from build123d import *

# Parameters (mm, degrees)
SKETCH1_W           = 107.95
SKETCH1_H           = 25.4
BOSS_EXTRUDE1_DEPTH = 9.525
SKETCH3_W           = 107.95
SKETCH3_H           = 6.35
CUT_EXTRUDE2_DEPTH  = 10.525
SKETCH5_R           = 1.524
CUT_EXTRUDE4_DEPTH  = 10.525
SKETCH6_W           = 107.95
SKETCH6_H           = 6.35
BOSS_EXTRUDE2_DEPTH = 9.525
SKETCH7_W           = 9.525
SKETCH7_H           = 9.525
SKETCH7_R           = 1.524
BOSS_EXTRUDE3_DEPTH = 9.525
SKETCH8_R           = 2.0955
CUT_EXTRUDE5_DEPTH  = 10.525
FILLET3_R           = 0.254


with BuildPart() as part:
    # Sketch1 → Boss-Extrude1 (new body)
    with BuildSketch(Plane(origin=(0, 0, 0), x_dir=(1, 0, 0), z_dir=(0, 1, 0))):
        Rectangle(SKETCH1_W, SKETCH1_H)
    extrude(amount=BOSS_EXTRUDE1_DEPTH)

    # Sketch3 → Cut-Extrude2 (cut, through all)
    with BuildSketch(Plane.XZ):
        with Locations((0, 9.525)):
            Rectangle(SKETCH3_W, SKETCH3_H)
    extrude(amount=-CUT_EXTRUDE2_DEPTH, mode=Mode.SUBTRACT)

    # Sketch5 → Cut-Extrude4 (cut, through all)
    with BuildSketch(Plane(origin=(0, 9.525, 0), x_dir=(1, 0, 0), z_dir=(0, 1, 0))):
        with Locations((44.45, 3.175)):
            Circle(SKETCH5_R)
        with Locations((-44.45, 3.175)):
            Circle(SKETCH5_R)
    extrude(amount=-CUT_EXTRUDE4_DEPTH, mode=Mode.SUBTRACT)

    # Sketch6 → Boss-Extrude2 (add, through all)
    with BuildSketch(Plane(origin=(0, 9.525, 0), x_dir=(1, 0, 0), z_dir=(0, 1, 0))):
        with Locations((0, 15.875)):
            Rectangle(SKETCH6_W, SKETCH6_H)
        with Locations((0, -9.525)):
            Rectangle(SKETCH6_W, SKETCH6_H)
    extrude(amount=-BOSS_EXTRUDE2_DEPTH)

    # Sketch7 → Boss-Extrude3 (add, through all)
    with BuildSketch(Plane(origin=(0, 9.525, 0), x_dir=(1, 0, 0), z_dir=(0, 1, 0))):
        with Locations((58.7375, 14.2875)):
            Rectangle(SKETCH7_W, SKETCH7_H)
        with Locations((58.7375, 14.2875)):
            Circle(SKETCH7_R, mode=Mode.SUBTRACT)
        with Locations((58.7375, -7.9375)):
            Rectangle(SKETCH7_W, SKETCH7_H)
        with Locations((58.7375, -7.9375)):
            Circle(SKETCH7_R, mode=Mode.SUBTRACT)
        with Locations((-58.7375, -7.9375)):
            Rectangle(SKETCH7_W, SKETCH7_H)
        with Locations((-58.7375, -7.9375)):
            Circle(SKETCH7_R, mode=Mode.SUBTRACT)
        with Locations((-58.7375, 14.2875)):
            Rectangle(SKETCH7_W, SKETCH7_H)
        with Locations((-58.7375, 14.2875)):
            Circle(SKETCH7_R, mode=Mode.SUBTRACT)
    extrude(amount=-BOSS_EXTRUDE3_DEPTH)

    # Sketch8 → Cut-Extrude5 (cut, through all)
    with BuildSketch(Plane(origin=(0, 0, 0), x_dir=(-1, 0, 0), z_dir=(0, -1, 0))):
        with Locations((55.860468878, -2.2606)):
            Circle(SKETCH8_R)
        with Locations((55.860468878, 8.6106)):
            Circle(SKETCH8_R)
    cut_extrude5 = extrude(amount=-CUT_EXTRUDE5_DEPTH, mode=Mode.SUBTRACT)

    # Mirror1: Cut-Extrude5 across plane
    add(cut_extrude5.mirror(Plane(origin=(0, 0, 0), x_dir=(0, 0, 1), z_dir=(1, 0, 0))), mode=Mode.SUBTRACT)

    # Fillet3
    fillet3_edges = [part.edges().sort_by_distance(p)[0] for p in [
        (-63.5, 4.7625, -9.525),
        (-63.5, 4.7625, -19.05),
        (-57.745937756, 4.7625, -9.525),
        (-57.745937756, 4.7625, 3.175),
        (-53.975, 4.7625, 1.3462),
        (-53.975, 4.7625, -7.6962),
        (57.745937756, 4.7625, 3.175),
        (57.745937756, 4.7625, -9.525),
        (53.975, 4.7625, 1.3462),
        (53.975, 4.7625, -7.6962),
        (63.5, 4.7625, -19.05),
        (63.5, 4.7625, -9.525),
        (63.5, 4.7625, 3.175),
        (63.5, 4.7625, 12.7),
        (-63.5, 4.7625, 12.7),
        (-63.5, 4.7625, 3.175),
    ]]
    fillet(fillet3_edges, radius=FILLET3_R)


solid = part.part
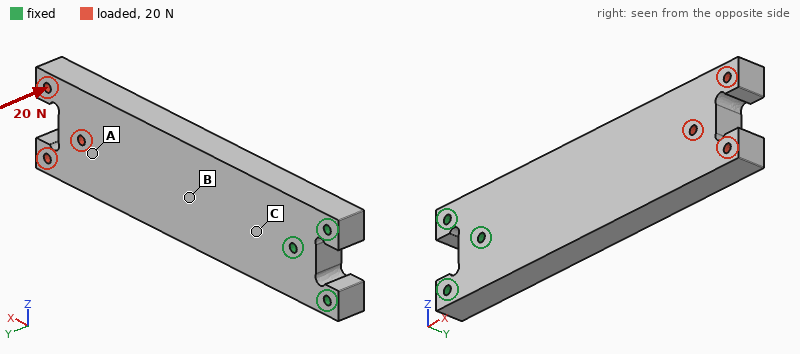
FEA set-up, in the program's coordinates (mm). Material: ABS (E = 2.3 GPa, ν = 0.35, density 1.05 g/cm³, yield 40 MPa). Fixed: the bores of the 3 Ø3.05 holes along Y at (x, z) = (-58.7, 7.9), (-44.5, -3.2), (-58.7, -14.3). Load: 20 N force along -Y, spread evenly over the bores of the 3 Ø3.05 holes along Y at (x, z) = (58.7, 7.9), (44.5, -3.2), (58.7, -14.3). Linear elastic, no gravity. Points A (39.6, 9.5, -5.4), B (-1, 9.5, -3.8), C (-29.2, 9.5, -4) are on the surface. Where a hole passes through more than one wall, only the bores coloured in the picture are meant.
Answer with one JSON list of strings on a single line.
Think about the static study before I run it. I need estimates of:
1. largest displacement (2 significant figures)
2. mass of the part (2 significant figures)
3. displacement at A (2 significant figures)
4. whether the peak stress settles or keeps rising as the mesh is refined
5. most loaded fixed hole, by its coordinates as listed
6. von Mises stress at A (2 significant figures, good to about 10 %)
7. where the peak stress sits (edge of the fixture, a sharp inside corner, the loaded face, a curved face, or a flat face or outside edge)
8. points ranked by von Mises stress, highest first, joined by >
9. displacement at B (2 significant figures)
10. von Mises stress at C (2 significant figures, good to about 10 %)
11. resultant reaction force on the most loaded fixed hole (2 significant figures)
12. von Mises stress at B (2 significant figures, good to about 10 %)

["1.5 mm", "37 g", "1.0 mm", "keeps rising", "(-44.5, -3.2)", "0.60 MPa", "edge of the fixture", "C > B > A", "0.36 mm", "3.3 MPa", "85 N", "2.3 MPa"]
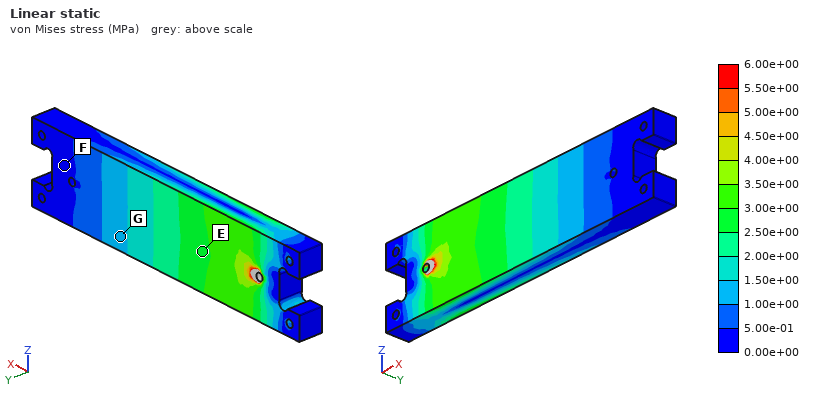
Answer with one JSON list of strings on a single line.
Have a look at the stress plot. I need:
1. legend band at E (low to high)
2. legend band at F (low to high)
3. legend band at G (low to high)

["2.50e+00 to 3.00e+00 MPa", "0.00e+00 to 5.00e-01 MPa", "1.00e+00 to 1.50e+00 MPa"]
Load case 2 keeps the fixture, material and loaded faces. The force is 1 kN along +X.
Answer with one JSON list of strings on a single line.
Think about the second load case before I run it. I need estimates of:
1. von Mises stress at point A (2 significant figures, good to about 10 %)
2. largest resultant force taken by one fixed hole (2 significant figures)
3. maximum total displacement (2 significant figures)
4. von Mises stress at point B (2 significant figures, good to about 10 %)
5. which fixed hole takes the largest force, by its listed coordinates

["3.6 MPa", "600 N", "0.17 mm", "3.3 MPa", "(-44.5, -3.2)"]
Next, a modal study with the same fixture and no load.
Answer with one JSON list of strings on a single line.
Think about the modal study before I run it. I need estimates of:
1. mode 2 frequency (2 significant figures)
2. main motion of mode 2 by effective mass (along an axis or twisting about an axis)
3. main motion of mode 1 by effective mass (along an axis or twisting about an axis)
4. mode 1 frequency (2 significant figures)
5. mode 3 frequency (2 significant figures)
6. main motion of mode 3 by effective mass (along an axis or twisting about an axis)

["540 Hz", "along Z", "along Y", "200 Hz", "1100 Hz", "twisting about X"]
